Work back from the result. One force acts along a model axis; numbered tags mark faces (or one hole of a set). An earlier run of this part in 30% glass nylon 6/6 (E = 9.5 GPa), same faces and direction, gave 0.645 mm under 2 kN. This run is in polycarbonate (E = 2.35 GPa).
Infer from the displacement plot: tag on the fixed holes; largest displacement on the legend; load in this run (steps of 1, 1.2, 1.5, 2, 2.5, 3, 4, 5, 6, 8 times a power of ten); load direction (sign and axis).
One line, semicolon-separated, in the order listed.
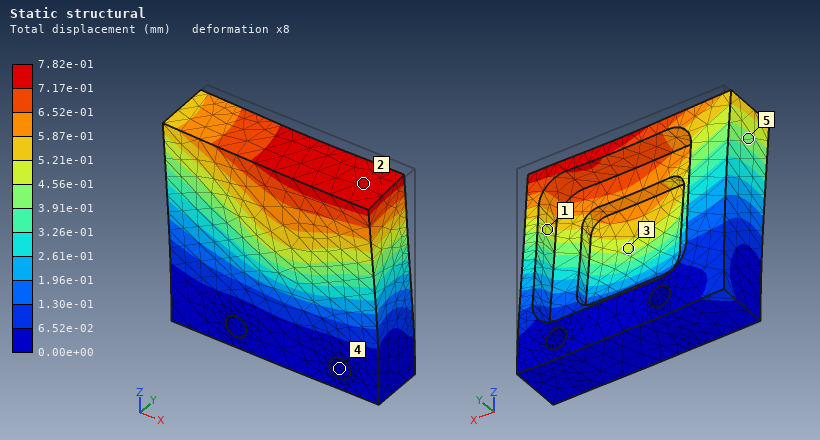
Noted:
4; 7.82e-01 mm; 600 N; -Y
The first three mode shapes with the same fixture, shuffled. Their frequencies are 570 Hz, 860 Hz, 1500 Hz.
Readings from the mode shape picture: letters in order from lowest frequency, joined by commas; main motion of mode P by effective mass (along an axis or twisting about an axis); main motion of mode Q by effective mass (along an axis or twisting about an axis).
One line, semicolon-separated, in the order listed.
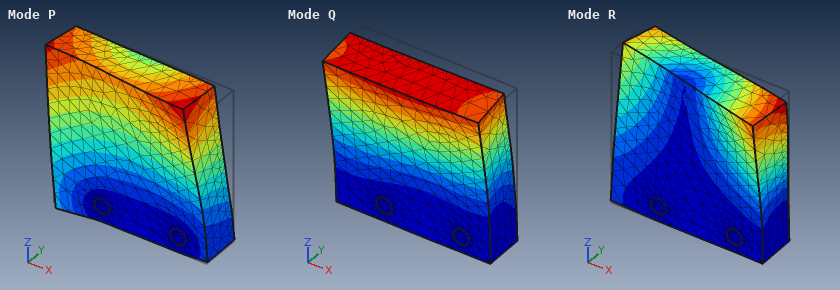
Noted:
Q, R, P; along X; along Y
